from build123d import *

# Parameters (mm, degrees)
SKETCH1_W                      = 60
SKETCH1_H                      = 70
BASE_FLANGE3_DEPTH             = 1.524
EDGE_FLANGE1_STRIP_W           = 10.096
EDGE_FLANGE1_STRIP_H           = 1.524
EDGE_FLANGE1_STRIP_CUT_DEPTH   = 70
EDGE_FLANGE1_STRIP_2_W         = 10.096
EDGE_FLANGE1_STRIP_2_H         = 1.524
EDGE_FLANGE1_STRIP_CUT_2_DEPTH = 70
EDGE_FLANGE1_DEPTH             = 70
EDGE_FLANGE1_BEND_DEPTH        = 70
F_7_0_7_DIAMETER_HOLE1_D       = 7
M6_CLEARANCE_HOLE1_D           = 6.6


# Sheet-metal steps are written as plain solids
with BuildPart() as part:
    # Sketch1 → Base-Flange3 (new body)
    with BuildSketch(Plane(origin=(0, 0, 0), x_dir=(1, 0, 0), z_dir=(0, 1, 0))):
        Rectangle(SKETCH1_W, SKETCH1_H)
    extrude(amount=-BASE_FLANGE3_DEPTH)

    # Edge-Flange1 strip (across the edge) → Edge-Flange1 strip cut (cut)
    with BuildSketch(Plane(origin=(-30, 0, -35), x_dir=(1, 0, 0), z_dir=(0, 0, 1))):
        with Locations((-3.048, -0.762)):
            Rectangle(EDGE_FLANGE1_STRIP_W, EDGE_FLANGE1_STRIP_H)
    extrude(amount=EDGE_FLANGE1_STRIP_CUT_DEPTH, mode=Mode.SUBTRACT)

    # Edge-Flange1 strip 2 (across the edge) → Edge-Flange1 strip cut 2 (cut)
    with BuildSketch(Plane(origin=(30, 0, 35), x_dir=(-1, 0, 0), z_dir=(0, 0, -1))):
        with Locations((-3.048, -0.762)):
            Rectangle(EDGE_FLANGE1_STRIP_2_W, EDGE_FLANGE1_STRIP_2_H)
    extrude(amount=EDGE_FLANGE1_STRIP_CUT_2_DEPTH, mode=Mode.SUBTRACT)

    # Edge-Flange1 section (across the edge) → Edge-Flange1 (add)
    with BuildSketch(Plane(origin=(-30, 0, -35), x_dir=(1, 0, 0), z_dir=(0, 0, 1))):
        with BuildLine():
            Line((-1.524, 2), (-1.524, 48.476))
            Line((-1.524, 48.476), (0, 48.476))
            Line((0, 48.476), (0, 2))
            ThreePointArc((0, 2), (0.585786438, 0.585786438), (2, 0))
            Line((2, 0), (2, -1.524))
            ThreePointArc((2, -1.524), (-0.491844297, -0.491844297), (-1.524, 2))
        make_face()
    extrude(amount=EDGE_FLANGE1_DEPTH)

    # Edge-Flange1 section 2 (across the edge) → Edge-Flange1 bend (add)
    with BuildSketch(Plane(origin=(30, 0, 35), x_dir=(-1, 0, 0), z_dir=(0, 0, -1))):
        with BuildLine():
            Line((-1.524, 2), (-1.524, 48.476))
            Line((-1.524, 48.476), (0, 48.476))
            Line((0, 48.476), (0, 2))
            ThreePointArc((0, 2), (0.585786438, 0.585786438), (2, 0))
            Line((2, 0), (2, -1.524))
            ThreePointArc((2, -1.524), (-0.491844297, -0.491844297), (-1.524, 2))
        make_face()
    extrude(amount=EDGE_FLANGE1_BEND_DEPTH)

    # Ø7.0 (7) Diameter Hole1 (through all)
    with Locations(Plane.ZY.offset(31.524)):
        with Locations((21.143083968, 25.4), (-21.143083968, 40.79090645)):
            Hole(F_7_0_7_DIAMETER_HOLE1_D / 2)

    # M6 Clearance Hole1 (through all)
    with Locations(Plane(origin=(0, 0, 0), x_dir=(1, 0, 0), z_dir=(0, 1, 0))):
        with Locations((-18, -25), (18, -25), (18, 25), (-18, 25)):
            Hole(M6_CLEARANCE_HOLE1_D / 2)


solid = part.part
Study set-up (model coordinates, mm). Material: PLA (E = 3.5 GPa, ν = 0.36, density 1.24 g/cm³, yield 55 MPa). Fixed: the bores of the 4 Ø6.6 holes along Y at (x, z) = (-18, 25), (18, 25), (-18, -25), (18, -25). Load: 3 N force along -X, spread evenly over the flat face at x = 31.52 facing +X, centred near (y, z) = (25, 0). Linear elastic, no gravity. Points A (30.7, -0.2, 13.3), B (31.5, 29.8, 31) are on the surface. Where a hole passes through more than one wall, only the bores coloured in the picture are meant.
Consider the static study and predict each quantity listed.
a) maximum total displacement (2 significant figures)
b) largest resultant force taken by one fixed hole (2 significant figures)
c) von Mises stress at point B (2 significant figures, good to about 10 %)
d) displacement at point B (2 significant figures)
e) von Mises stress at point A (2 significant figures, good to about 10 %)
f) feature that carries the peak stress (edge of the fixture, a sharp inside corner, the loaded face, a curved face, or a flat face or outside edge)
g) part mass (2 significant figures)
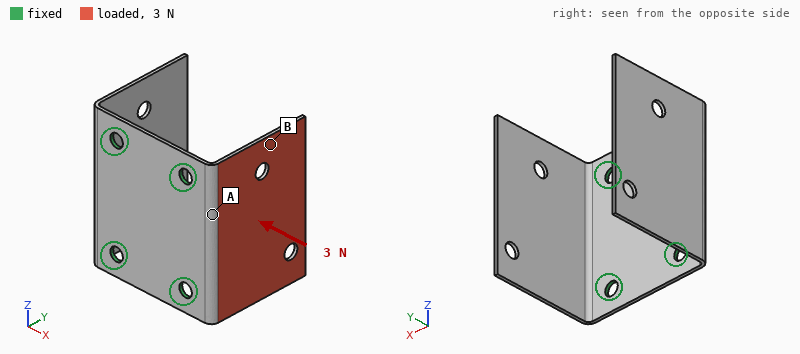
1.1 mm
1.1 N
0.51 MPa
0.61 mm
2.2 MPa
a flat face or outside edge
20 g
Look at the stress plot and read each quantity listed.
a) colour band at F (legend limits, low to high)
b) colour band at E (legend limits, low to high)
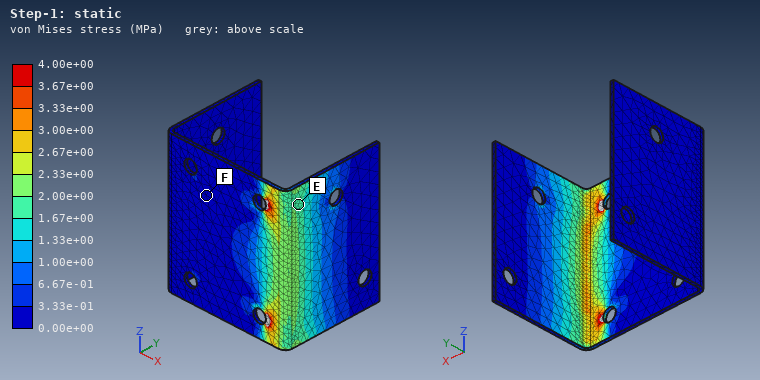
0.00e+00 to 3.33e-01 MPa
1.67e+00 to 2.00e+00 MPa
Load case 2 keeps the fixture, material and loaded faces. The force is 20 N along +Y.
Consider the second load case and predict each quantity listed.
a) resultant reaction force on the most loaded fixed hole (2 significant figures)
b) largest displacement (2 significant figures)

11 N
1.1 mm
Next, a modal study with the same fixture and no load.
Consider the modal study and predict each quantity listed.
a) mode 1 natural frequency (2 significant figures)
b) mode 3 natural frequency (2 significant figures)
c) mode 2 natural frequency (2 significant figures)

130 Hz
280 Hz
130 Hz
